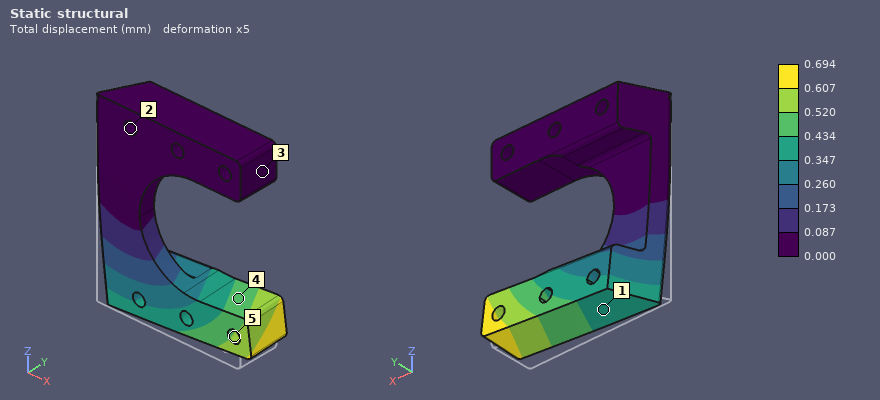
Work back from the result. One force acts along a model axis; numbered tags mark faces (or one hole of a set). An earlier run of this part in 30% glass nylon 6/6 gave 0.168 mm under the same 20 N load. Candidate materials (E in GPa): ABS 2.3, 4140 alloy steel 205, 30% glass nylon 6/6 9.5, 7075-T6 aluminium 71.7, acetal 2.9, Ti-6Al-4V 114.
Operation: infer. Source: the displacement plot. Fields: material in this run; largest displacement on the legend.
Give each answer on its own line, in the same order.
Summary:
ABS
0.694 mm
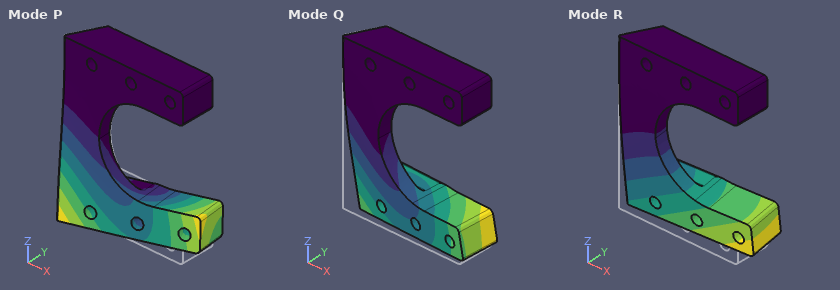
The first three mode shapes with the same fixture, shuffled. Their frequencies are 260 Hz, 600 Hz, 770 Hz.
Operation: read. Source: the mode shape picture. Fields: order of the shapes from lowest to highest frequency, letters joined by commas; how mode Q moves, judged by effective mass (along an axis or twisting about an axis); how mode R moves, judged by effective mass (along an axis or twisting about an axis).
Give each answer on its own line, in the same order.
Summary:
R, Q, P
along X
along Y
